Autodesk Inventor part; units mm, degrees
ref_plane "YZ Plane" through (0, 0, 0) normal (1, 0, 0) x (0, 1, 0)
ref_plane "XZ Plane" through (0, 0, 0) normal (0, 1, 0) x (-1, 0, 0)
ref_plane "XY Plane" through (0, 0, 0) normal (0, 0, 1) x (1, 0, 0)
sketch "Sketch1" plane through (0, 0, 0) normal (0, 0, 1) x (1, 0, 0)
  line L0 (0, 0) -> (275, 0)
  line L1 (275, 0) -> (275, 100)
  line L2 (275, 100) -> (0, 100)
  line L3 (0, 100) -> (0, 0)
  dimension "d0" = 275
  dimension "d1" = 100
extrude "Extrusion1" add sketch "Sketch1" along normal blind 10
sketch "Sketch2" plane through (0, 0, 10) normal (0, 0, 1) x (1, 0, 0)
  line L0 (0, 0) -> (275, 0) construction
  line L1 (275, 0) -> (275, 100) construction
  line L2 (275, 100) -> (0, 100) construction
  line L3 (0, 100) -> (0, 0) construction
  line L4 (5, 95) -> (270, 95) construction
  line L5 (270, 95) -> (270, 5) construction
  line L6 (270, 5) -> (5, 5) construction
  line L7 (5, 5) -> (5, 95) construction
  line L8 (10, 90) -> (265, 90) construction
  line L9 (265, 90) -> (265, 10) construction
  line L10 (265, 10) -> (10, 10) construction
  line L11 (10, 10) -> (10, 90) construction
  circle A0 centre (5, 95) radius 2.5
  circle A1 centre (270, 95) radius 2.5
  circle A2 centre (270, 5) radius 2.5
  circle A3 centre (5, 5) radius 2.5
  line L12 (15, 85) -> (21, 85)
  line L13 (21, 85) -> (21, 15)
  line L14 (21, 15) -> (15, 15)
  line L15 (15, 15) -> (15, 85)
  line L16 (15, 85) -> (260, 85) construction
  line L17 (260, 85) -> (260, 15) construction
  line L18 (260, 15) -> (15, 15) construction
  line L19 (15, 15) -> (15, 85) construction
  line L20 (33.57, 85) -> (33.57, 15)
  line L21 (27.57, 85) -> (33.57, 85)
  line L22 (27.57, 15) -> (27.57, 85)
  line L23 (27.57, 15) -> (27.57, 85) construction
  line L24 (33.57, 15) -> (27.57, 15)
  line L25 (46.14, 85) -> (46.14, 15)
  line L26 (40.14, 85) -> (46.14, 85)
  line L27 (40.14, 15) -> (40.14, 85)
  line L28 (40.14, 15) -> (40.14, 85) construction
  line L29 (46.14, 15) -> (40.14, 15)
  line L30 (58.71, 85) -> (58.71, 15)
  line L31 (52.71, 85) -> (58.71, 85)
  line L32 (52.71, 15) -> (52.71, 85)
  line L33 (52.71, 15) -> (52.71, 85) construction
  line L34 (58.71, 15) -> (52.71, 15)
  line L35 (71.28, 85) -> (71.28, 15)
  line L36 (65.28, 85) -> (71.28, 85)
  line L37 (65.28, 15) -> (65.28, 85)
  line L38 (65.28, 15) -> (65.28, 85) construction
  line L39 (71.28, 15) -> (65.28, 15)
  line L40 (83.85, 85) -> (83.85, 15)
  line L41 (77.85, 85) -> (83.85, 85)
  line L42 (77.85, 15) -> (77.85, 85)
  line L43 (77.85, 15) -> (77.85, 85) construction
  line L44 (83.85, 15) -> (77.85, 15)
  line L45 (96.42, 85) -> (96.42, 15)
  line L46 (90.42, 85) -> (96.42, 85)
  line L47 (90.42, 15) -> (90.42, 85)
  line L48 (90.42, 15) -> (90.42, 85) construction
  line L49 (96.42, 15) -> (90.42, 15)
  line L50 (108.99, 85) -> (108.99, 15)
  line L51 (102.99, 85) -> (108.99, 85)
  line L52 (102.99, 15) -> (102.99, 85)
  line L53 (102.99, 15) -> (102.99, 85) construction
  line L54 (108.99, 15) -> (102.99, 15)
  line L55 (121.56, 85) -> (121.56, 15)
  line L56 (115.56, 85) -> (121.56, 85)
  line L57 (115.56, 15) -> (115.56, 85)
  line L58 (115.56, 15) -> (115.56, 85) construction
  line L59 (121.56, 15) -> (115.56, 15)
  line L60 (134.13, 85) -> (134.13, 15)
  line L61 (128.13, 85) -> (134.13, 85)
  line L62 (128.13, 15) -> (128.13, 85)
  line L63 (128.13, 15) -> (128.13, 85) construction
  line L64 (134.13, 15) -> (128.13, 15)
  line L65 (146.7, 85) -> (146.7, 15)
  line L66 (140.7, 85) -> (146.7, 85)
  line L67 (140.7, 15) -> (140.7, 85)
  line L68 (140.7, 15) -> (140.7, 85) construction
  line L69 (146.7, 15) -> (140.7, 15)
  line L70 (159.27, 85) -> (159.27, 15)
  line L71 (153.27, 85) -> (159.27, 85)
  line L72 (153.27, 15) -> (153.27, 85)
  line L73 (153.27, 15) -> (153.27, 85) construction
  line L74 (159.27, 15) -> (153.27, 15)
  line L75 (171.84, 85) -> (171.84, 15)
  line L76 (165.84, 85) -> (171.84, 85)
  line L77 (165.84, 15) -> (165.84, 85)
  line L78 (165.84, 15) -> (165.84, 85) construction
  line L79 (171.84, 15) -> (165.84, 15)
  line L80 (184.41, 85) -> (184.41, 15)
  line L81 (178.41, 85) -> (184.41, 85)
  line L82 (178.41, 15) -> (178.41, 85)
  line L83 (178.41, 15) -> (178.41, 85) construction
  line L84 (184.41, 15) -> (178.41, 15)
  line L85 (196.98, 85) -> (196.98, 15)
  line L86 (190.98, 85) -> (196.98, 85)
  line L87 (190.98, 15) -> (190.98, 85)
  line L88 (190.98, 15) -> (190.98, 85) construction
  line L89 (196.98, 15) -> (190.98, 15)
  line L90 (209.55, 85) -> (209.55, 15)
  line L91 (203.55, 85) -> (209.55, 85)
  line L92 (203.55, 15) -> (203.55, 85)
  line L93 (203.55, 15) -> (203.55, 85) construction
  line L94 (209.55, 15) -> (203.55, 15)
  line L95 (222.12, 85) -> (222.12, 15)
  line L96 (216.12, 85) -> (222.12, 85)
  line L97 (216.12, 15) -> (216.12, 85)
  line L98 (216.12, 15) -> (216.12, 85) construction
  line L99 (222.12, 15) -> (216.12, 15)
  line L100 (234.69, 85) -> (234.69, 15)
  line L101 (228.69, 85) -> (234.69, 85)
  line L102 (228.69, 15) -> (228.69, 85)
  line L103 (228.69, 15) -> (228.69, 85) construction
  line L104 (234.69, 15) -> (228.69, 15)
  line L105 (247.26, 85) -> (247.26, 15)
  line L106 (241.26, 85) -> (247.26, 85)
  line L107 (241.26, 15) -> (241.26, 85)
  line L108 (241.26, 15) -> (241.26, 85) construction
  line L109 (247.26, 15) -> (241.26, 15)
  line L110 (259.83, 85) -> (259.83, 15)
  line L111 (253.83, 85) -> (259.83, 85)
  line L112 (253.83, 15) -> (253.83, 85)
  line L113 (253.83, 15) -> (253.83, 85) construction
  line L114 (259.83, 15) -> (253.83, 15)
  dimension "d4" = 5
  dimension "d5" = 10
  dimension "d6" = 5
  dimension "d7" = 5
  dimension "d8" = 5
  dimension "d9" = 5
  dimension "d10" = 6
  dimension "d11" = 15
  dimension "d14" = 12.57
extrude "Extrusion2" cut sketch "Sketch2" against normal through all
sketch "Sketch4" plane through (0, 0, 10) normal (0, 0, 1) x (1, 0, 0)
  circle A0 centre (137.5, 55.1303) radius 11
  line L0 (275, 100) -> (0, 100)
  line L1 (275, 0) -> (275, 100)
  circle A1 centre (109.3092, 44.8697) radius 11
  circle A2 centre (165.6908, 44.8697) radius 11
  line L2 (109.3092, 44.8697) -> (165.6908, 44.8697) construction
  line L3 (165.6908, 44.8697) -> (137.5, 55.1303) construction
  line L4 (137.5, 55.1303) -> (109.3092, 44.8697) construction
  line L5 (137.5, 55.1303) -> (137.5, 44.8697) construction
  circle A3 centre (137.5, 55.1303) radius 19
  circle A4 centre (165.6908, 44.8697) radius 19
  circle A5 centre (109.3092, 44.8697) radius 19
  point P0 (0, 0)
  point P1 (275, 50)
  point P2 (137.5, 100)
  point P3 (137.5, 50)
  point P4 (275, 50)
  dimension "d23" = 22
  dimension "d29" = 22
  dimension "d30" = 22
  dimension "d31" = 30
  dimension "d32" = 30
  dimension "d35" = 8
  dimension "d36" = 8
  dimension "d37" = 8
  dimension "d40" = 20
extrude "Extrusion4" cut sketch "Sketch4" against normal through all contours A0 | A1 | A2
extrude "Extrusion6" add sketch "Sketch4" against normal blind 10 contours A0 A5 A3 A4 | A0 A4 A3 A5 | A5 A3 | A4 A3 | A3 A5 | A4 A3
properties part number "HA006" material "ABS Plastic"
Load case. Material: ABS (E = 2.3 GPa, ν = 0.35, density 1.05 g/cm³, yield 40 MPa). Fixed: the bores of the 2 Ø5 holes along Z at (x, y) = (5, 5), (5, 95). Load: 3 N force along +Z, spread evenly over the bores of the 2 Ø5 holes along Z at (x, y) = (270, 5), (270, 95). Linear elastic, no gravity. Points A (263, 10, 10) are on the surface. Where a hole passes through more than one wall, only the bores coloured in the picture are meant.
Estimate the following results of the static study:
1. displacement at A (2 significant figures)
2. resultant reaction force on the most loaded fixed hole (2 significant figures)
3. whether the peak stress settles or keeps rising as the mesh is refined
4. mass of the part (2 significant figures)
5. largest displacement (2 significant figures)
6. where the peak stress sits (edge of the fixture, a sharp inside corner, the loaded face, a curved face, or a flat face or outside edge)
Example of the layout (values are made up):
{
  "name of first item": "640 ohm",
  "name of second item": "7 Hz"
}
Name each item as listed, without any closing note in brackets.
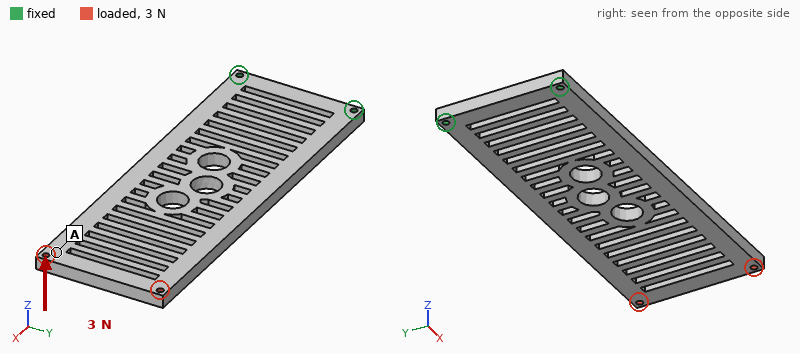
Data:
{
  "displacement at A": "2.8 mm",
  "resultant reaction force on the most loaded fixed hole": "1.5 N",
  "whether the peak stress settles or keeps rising as the mesh is refined": "keeps rising",
  "mass of the part": "200 g",
  "largest displacement": "3.0 mm",
  "where the peak stress sits": "edge of the fixture"
}
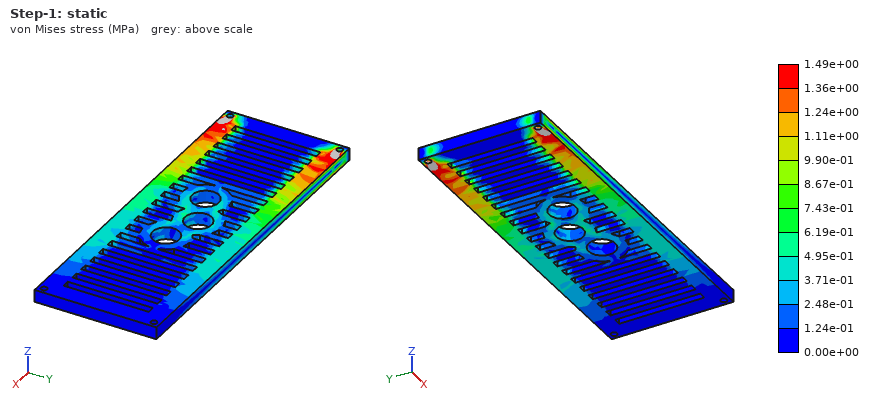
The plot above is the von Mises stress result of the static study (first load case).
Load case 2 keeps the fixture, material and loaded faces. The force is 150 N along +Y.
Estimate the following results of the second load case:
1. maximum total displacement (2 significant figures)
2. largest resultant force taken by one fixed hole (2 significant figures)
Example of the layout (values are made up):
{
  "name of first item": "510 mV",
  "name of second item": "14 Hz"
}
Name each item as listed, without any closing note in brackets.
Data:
{
  "maximum total displacement": "2.0 mm",
  "largest resultant force taken by one fixed hole": "430 N"
}
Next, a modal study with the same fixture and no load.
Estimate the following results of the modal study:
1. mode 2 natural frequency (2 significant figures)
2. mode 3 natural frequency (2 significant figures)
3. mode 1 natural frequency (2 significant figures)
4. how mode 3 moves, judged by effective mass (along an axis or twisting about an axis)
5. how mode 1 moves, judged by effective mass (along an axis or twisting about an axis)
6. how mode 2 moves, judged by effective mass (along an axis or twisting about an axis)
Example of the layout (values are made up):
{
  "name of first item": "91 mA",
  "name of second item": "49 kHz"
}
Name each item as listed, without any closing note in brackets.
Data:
{
  "mode 2 natural frequency": "130 Hz",
  "mode 3 natural frequency": "140 Hz",
  "mode 1 natural frequency": "22 Hz",
  "how mode 3 moves, judged by effective mass": "along Z",
  "how mode 1 moves, judged by effective mass": "along Z",
  "how mode 2 moves, judged by effective mass": "twisting about X"
}
